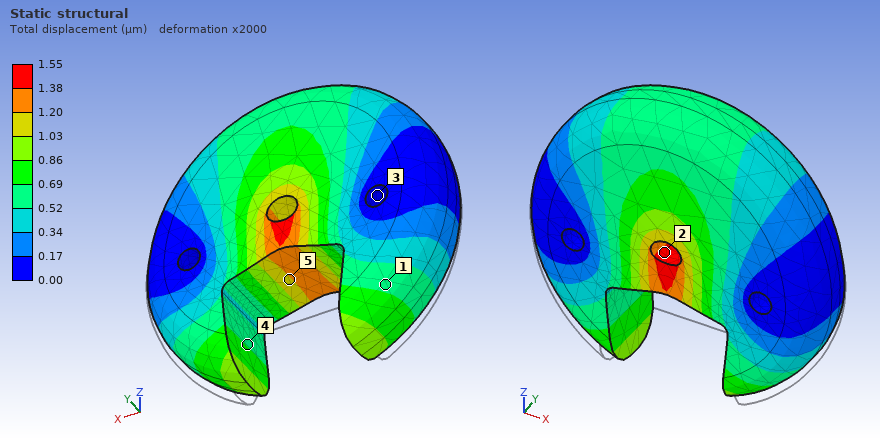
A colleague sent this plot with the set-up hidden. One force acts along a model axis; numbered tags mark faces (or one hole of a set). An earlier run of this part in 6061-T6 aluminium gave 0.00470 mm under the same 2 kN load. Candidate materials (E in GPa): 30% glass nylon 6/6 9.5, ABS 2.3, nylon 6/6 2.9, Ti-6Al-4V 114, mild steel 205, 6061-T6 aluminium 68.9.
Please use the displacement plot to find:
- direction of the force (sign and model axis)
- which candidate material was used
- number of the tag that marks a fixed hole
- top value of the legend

+Z
mild steel
3
1.55 µm
